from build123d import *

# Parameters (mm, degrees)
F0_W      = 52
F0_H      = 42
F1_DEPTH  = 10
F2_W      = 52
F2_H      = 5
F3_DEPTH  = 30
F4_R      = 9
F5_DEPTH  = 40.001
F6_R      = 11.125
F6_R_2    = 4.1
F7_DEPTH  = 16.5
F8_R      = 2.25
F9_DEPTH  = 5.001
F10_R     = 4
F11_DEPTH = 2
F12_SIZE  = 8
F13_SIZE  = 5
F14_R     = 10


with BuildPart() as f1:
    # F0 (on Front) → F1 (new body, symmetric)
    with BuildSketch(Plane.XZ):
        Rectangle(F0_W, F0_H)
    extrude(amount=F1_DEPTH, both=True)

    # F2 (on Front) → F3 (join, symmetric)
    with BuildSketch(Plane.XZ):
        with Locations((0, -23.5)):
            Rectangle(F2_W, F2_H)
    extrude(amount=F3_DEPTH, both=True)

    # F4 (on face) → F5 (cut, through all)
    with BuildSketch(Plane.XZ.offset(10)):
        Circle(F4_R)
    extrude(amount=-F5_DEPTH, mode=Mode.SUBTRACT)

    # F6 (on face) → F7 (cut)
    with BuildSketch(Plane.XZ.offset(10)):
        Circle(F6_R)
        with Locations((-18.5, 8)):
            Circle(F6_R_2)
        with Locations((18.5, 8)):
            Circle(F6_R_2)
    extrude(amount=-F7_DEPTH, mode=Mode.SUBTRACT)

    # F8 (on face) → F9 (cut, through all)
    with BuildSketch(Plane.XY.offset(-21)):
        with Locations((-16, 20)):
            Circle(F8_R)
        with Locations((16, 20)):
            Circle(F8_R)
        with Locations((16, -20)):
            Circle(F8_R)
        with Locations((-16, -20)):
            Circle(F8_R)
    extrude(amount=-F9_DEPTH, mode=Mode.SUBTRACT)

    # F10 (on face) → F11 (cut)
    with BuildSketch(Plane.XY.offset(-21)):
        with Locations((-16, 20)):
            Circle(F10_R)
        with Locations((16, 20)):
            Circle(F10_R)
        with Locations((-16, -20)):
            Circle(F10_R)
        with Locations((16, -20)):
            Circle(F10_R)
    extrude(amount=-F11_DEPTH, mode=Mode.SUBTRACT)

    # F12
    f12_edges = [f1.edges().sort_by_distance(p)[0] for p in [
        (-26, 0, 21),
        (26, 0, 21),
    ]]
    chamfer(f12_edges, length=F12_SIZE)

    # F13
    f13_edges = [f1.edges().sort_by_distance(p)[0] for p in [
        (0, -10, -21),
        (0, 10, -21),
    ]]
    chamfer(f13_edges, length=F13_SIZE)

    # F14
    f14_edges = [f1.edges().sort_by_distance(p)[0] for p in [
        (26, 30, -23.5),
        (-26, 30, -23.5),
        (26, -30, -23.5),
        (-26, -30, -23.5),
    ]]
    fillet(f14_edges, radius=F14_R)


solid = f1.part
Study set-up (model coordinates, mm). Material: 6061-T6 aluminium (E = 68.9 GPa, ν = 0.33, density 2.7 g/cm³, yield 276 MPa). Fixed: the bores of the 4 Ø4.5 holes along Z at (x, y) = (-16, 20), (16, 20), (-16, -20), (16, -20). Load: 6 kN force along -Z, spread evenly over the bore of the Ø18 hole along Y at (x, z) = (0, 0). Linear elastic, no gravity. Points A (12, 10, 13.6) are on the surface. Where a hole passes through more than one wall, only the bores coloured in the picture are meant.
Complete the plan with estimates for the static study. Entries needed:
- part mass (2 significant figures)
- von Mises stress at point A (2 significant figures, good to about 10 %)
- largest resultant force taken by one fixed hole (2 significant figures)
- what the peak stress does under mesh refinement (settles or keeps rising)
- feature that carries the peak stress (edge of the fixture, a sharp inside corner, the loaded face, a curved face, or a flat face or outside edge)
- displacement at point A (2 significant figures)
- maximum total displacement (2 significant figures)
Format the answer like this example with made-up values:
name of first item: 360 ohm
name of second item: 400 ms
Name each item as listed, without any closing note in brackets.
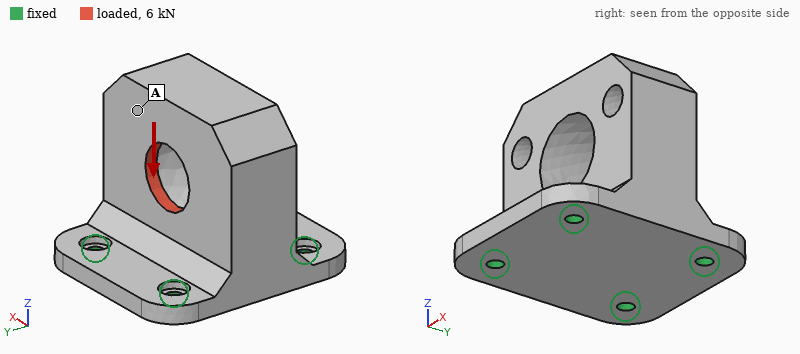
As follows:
part mass: 130 g
von Mises stress at point A: 17 MPa
largest resultant force taken by one fixed hole: 2.5 kN
what the peak stress does under mesh refinement: keeps rising
feature that carries the peak stress: edge of the fixture
displacement at point A: 41 µm
maximum total displacement: 50 µm
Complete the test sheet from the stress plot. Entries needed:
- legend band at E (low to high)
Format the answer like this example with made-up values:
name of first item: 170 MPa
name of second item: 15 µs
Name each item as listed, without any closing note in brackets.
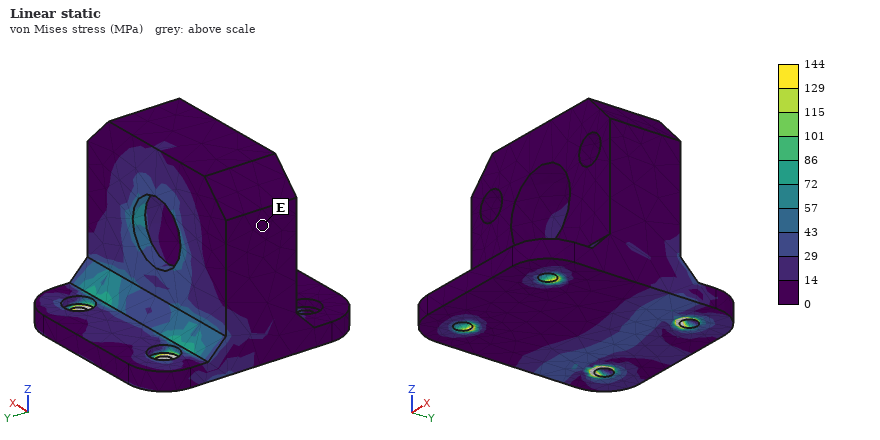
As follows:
legend band at E: 0 to 14 MPa
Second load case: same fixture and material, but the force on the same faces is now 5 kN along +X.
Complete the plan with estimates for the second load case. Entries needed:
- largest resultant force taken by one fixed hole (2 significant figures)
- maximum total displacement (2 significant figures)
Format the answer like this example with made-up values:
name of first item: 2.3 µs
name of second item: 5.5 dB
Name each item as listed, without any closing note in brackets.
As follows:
largest resultant force taken by one fixed hole: 2.9 kN
maximum total displacement: 86 µm
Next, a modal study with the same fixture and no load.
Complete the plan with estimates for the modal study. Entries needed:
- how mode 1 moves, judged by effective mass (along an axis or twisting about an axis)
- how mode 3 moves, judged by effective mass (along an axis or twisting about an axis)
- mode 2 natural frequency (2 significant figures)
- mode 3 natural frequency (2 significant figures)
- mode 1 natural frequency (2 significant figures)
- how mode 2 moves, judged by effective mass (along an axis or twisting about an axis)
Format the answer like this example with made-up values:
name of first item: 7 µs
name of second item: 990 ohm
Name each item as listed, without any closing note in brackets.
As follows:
how mode 1 moves, judged by effective mass: along X
how mode 3 moves, judged by effective mass: along Z
mode 2 natural frequency: 5300 Hz
mode 3 natural frequency: 8600 Hz
mode 1 natural frequency: 4600 Hz
how mode 2 moves, judged by effective mass: along Y
